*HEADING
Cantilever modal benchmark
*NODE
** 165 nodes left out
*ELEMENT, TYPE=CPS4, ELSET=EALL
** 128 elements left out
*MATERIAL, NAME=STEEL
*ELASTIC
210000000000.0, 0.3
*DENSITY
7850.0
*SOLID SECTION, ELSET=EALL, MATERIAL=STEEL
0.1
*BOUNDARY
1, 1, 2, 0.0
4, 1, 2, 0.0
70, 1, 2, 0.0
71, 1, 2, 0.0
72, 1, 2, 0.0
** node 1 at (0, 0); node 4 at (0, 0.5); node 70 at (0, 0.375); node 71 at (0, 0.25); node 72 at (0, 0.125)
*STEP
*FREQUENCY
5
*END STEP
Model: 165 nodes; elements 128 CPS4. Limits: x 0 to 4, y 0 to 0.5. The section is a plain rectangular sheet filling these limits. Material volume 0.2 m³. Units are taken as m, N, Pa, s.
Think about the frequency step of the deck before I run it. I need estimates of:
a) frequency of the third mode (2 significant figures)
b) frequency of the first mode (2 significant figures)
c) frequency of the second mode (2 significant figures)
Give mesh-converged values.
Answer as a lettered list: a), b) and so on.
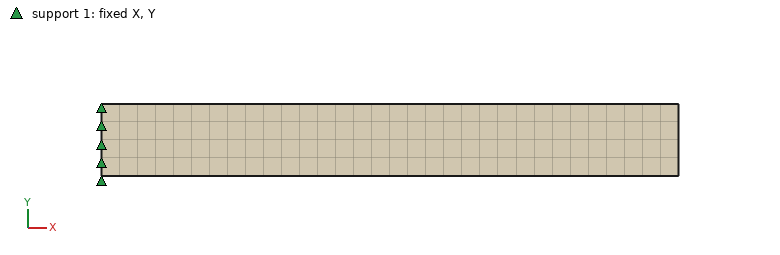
a) 320 Hz
b) 26 Hz
c) 150 Hz
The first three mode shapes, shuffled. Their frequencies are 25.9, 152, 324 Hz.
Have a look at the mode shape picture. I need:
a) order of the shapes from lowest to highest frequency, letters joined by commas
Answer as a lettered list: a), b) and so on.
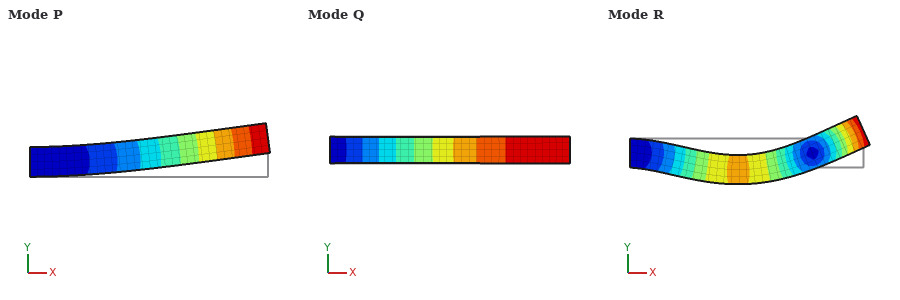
a) P, R, Q
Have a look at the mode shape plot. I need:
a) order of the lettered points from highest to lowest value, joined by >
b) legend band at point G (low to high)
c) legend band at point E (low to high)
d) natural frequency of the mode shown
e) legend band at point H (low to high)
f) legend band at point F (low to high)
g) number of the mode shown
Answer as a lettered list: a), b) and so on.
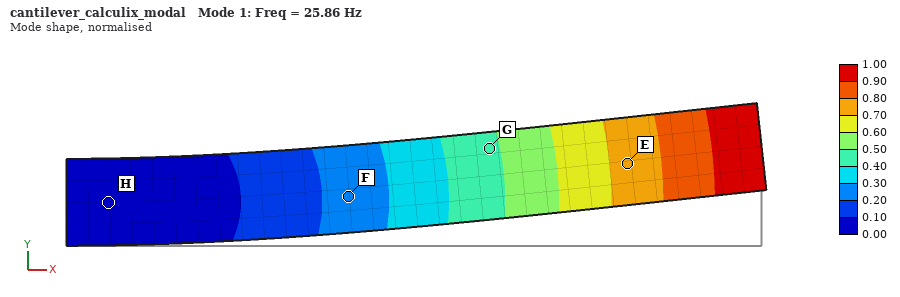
a) E > G > F > H
b) 0.40 to 0.50
c) 0.70 to 0.80
d) 25.86 Hz
e) 0.00 to 0.10
f) 0.20 to 0.30
g) 1
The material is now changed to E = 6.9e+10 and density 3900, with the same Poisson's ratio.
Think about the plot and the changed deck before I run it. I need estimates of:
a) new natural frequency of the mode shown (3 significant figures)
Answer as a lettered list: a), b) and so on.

a) 21.0 Hz
